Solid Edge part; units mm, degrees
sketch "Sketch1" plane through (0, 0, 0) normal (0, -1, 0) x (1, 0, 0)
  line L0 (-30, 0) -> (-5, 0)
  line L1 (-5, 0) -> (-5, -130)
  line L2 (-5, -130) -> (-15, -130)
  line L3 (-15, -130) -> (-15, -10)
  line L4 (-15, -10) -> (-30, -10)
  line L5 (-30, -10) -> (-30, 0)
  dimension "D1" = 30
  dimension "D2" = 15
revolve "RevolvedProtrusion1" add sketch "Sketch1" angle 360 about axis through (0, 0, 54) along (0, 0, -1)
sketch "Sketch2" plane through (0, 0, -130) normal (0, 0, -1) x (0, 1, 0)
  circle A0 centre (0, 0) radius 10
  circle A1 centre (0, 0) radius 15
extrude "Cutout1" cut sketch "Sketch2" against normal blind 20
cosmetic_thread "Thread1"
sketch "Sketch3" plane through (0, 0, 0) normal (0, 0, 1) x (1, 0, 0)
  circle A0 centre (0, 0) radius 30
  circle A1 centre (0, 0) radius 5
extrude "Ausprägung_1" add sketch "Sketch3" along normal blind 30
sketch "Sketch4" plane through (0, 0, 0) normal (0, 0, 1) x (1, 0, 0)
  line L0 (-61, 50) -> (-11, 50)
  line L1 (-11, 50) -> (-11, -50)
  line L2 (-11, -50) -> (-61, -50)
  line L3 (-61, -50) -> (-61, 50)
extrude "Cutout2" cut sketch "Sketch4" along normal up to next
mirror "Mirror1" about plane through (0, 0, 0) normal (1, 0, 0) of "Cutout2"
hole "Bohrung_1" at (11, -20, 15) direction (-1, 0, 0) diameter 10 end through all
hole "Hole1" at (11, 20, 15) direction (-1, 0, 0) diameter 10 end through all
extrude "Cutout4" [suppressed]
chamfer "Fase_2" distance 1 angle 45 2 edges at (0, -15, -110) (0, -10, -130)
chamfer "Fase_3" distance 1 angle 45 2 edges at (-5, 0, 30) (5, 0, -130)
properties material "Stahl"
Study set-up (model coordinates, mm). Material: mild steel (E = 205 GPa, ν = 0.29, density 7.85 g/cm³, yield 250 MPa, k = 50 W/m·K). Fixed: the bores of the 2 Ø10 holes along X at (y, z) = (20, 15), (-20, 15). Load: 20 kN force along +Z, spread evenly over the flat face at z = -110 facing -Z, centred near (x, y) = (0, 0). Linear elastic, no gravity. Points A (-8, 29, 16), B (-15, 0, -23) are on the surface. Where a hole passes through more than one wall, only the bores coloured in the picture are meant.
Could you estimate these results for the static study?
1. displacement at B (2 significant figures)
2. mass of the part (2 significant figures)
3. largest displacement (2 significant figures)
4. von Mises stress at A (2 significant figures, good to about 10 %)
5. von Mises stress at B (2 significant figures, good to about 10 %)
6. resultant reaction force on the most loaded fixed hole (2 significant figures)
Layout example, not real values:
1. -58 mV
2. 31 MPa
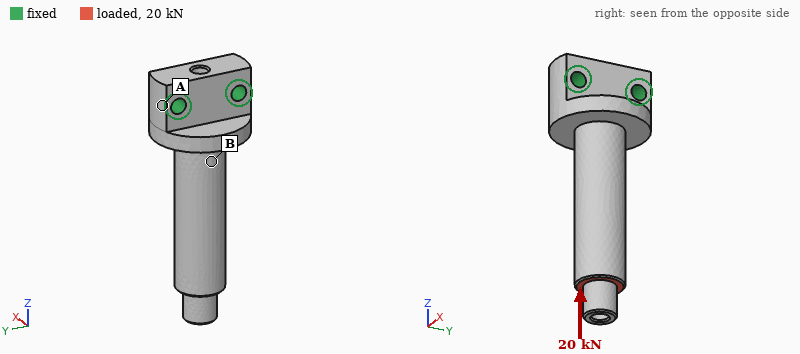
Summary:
1. 5.4 µm
2. 1.0 kg
3. 19 µm
4. 6.7 MPa
5. 30 MPa
6. 11 kN
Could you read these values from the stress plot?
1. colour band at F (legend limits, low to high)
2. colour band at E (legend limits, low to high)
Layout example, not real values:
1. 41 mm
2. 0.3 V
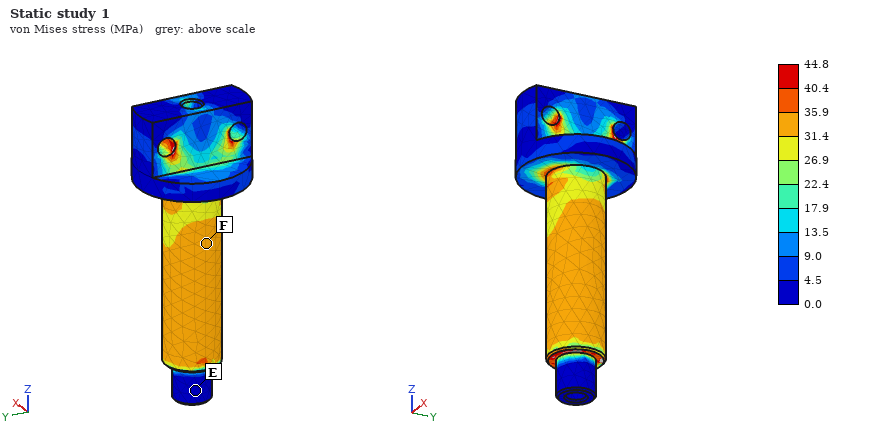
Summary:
1. 31.4 to 35.9 MPa
2. 0.0 to 4.5 MPa
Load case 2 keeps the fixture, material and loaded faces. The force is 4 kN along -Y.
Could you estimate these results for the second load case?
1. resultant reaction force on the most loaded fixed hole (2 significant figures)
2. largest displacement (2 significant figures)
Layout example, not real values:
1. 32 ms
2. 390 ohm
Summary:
1. 12 kN
2. 0.28 mm
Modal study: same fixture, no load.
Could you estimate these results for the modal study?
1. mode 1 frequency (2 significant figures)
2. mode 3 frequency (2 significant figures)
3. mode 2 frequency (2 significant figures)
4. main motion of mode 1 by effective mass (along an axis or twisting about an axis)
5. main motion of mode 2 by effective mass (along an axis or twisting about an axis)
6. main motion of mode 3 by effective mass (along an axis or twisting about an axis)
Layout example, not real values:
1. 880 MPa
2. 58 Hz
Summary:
1. 1300 Hz
2. 6400 Hz
3. 1600 Hz
4. along X
5. along Y
6. along X
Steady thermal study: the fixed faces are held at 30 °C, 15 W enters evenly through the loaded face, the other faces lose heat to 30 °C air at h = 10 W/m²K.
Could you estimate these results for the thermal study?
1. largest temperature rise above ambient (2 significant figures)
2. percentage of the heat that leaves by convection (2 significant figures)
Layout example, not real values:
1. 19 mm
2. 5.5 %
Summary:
1. 45 K
2. 28 %
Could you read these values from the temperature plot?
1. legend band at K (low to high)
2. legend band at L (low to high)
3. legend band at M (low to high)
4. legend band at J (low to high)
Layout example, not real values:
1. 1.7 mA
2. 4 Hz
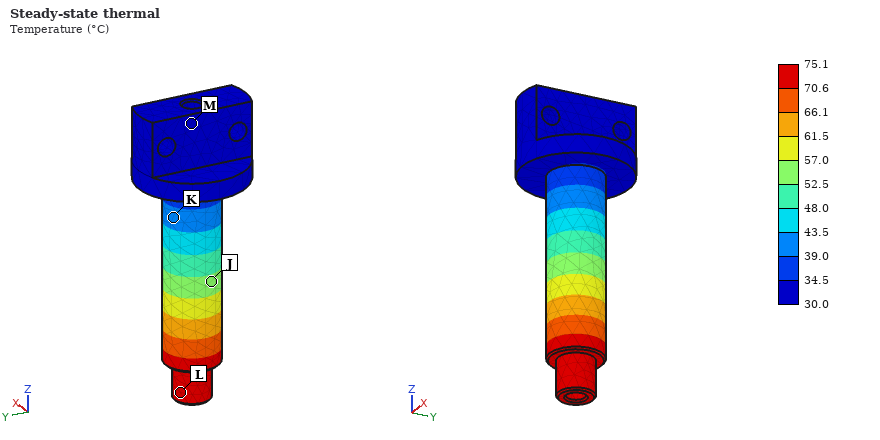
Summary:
1. 39.0 to 43.5 °C
2. 70.6 to 75.1 °C
3. 30.0 to 34.5 °C
4. 52.5 to 57.0 °C
